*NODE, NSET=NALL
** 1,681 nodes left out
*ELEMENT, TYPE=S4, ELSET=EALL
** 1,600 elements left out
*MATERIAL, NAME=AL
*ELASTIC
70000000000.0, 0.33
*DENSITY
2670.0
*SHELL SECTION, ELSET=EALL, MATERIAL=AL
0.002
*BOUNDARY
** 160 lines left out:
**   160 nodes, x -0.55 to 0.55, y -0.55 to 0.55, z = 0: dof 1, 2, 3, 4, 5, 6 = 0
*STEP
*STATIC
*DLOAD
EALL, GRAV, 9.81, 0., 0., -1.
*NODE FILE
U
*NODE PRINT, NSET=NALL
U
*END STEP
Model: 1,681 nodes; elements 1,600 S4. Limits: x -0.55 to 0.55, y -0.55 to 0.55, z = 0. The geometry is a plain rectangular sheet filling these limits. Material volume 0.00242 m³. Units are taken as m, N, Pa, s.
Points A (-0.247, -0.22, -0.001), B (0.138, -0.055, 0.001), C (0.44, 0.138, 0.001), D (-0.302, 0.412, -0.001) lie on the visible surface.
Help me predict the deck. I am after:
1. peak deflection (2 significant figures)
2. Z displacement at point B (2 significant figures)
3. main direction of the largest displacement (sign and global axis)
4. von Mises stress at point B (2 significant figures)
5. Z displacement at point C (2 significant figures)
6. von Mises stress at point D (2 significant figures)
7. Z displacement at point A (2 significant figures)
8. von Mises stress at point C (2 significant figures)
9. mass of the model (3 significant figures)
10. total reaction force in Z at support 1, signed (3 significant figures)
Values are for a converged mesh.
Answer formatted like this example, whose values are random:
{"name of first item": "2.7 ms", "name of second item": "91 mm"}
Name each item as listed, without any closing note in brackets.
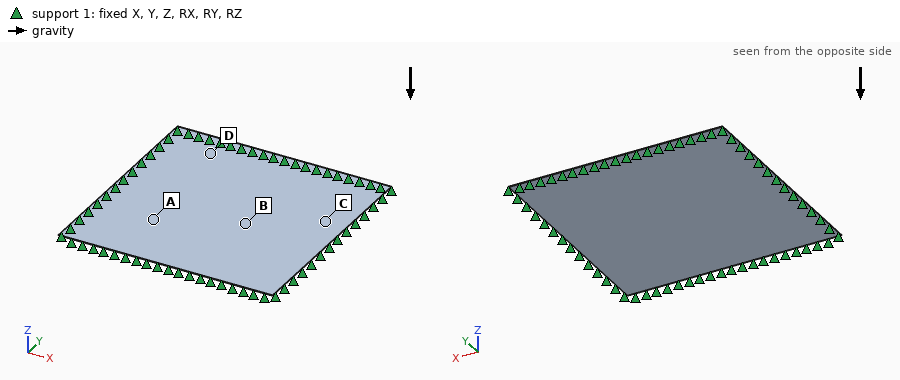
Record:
{"peak deflection": "0.0018 m", "Z displacement at point B": "-0.0016 m", "main direction of the largest displacement": "-Z", "von Mises stress at point B": "1.9e+06 Pa", "Z displacement at point C": "-2.4e-04 m", "von Mises stress at point D": "1.3e+06 Pa", "Z displacement at point A": "-9.0e-04 m", "von Mises stress at point C": "1.4e+06 Pa", "mass of the model": "6.46 kg", "total reaction force in Z at support 1, signed": "63.4 N"}
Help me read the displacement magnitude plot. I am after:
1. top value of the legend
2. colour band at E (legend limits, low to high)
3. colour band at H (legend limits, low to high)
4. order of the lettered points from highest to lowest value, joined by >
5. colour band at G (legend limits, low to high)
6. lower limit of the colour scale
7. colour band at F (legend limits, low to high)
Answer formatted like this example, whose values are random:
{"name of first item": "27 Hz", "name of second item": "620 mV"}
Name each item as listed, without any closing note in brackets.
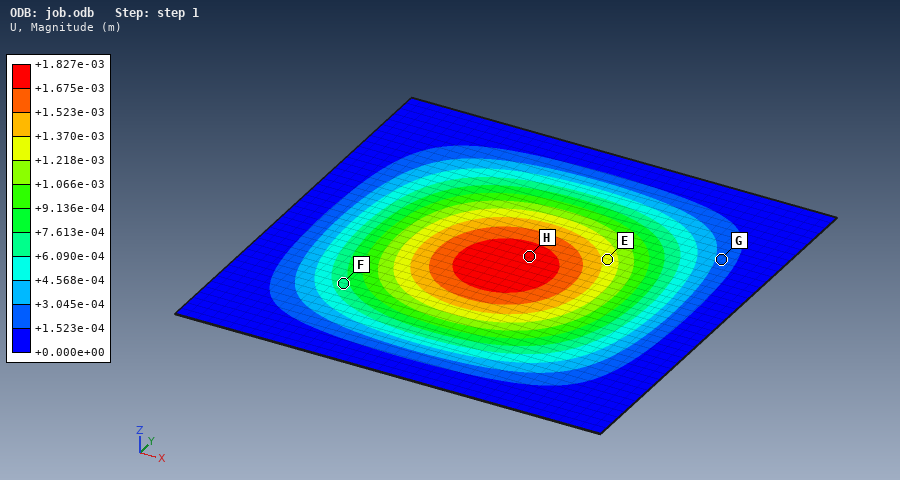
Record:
{"top value of the legend": "+1.827e-03 m", "colour band at E": "+1.218e-03 to +1.370e-03 m", "colour band at H": "+1.675e-03 to +1.827e-03 m", "order of the lettered points from highest to lowest value, joined by >": "H > E > F > G", "colour band at G": "+1.523e-04 to +3.045e-04 m", "lower limit of the colour scale": "+0.000e+00 m", "colour band at F": "+6.090e-04 to +7.613e-04 m"}
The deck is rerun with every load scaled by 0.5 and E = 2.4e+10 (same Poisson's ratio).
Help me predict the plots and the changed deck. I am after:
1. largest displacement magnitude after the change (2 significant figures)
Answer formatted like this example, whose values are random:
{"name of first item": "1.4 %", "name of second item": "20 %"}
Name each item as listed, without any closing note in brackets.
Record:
{"largest displacement magnitude after the change": "0.0027 m"}
